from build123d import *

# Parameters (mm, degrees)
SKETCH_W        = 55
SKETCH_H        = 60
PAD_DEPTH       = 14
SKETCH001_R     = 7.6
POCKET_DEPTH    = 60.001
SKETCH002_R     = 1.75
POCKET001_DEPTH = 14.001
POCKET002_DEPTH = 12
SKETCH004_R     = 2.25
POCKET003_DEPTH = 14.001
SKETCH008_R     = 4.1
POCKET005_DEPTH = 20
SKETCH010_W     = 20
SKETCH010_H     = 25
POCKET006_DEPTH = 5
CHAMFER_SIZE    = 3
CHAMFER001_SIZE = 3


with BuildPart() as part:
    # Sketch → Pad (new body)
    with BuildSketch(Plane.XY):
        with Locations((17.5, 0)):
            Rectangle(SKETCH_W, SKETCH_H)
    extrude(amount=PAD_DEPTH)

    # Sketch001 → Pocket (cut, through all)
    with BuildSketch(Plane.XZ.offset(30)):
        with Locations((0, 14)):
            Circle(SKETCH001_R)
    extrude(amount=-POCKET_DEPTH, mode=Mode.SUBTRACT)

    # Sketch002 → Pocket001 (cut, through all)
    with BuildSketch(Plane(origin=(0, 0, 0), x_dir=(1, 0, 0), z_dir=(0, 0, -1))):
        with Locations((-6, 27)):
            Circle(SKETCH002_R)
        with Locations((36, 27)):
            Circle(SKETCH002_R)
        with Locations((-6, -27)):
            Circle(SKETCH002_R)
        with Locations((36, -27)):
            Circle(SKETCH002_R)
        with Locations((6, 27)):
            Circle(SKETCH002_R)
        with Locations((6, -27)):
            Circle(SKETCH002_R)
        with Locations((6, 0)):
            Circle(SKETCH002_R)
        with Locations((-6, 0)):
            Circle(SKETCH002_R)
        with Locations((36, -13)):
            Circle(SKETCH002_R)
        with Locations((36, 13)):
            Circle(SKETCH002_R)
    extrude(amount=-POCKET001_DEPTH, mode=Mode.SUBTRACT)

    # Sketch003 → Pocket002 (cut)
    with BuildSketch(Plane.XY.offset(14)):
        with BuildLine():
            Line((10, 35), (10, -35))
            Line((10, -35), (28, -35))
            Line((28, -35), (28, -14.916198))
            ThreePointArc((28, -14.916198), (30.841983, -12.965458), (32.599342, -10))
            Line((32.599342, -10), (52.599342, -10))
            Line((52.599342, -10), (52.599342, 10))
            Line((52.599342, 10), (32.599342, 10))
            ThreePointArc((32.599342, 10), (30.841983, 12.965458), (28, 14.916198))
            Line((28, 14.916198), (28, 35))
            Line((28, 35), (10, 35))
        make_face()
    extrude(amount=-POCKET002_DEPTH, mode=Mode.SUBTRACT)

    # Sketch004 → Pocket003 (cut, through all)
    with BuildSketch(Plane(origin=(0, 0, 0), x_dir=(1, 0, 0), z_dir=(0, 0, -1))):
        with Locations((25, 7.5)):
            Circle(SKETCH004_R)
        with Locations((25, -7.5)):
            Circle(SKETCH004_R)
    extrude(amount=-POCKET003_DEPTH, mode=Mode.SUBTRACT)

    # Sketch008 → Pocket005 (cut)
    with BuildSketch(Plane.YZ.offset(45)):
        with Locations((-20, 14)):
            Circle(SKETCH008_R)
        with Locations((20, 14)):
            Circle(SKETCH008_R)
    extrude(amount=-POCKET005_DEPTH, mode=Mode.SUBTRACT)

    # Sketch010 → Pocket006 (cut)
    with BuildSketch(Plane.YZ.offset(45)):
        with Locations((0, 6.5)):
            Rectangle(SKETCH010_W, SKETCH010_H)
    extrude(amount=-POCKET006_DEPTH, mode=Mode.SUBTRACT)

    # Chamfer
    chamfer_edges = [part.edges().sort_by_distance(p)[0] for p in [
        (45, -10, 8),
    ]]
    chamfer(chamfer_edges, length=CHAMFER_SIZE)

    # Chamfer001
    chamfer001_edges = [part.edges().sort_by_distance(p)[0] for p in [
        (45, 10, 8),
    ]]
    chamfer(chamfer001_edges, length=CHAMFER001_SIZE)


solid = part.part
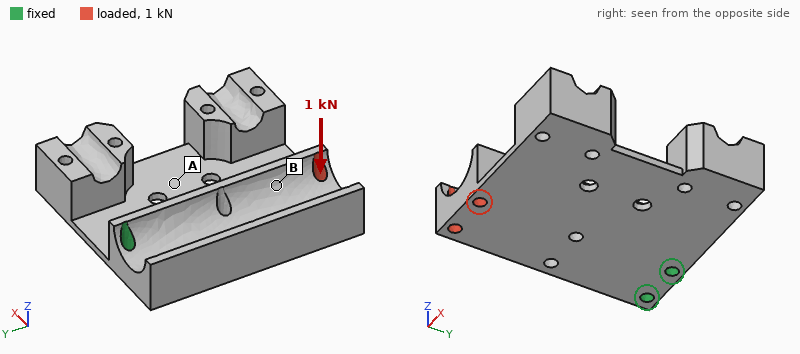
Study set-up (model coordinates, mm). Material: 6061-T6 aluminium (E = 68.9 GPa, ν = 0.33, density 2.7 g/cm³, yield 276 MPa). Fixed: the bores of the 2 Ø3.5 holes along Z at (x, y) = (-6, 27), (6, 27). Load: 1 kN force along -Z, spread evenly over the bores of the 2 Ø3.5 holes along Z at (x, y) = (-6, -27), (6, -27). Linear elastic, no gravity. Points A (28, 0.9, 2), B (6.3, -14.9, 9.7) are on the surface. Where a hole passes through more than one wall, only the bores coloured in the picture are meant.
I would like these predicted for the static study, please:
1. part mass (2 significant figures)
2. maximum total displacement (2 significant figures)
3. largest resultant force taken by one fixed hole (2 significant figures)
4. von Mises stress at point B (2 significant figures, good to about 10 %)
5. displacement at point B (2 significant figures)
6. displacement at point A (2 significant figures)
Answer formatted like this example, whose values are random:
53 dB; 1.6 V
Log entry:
57 g; 0.38 mm; 600 N; 33 MPa; 0.23 mm; 0.089 mm
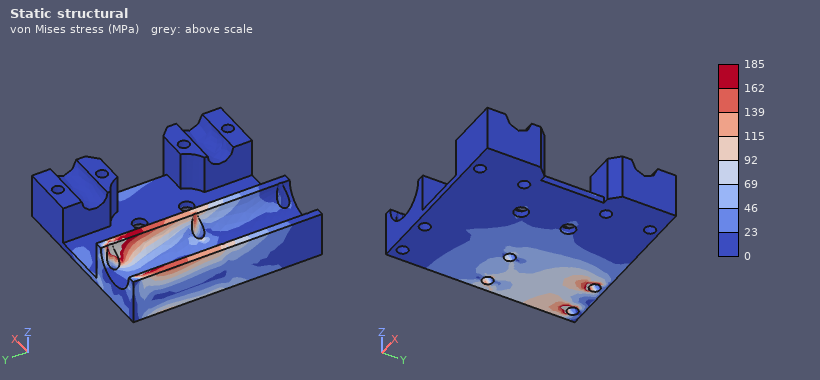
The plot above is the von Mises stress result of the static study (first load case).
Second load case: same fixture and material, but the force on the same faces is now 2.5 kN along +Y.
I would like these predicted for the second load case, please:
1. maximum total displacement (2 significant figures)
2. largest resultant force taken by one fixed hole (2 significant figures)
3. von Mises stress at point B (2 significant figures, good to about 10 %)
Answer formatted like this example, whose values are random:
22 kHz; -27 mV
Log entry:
16 µm; 1.3 kN; 13 MPa
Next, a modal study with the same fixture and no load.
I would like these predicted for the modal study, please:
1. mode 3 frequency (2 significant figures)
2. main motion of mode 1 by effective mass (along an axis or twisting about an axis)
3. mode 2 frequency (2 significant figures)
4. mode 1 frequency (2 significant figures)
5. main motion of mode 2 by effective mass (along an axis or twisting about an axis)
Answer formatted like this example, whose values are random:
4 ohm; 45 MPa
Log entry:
2400 Hz; along Z; 980 Hz; 610 Hz; twisting about X
